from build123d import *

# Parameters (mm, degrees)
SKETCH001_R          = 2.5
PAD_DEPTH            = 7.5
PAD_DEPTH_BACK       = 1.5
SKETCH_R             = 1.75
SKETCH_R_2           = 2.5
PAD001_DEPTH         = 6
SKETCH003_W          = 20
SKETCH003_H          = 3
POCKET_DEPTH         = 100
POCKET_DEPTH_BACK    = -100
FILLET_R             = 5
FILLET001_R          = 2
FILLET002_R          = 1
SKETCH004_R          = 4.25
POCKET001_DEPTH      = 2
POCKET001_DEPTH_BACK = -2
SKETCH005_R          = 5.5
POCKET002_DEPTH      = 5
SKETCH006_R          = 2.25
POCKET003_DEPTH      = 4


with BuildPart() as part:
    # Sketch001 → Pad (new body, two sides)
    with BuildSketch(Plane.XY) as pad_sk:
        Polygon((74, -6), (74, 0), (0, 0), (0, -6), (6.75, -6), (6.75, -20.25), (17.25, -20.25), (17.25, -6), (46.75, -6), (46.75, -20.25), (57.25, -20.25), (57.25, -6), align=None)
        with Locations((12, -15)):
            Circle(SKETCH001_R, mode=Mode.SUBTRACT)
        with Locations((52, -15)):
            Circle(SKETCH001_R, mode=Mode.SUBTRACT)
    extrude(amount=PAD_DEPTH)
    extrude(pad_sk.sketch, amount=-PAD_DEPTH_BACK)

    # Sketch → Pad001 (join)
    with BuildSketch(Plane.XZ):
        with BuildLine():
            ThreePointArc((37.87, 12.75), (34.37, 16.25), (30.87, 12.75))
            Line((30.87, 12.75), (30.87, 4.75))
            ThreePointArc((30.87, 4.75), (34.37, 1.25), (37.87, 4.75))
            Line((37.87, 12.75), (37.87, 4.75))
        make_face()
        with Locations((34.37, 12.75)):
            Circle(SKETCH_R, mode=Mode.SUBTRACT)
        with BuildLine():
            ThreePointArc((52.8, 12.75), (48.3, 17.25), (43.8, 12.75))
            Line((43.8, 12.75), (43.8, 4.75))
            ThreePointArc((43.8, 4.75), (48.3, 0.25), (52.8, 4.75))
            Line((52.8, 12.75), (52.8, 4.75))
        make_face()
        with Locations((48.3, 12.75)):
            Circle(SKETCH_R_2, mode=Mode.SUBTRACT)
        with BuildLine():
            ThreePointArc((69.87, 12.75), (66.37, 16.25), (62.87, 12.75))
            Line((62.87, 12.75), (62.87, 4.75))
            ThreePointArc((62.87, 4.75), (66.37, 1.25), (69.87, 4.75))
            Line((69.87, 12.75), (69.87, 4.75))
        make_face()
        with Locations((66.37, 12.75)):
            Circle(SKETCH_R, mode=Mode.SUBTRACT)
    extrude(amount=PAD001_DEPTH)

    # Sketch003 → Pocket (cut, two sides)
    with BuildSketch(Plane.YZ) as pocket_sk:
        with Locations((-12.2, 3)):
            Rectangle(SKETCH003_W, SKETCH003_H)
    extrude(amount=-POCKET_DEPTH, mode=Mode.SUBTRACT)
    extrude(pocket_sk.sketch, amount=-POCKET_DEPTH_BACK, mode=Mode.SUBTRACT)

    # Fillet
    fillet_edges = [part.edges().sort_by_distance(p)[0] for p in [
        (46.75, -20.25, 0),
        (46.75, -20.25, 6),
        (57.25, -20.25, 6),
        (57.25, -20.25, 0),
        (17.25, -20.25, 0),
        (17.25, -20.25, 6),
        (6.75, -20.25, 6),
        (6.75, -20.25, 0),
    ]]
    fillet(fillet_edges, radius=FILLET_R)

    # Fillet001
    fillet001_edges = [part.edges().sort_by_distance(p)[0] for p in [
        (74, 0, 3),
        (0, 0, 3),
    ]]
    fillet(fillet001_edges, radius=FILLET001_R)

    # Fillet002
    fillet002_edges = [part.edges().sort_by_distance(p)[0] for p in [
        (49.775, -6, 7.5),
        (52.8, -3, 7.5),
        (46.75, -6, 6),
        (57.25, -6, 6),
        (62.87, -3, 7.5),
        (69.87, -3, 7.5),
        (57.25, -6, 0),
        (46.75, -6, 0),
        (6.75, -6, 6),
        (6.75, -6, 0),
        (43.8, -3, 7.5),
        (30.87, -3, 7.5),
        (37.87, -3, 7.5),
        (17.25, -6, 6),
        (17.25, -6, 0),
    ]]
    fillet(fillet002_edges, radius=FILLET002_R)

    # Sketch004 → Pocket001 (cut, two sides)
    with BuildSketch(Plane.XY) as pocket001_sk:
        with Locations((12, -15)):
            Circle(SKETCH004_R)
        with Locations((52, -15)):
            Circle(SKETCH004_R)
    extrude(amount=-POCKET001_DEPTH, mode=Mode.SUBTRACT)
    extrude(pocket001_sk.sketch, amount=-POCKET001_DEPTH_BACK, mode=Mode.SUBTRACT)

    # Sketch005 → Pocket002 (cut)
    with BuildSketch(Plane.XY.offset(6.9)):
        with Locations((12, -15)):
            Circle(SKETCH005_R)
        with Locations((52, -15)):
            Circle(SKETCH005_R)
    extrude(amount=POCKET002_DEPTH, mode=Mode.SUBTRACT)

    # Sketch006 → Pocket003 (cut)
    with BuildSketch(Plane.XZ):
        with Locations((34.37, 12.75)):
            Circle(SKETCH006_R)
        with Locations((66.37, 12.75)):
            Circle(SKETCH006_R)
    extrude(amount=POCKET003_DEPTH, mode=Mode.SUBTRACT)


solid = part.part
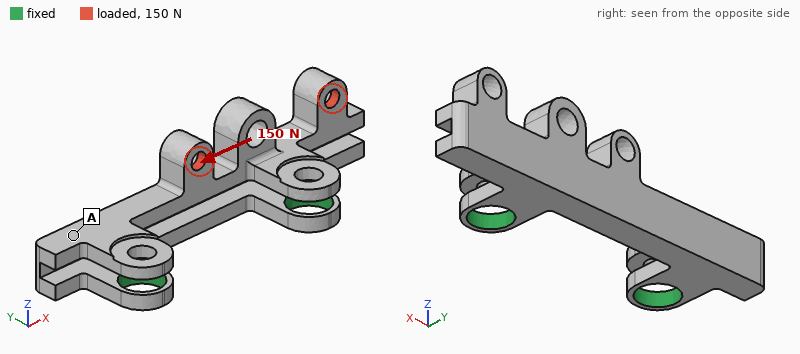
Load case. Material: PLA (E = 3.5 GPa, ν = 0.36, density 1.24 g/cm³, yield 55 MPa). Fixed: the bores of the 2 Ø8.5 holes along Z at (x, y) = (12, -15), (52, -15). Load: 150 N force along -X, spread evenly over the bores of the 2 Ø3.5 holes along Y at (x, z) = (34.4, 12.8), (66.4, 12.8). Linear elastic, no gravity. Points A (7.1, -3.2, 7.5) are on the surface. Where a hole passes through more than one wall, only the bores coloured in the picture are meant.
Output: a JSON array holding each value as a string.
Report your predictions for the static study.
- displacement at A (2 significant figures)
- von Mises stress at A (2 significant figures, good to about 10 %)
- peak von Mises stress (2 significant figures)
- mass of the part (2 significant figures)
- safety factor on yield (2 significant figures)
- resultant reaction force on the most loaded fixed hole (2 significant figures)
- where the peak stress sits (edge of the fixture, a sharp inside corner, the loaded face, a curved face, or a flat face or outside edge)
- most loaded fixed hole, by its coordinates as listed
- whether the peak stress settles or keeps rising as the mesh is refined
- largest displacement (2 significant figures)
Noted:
["0.18 mm", "3.2 MPa", "35 MPa", "6.4 g", "1.6", "93 N", "a curved face", "(12, -15)", "settles", "0.65 mm"]
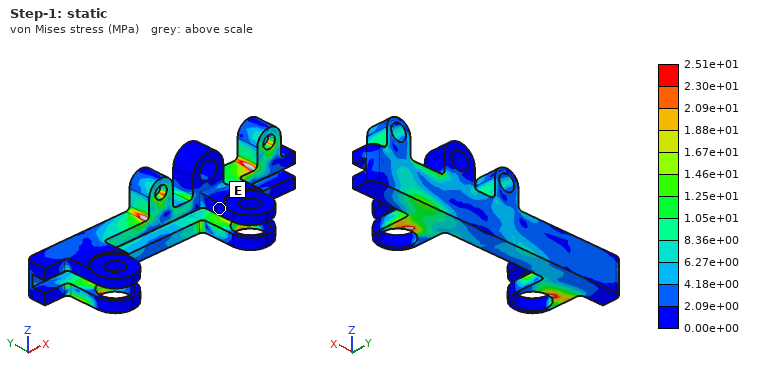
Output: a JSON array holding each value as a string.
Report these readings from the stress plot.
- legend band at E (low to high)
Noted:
["0.00e+00 to 2.09e+00 MPa"]
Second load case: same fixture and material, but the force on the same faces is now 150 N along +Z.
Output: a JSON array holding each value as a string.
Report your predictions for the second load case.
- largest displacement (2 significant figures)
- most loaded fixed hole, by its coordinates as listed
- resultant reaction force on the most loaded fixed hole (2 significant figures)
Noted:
["0.66 mm", "(52, -15)", "140 N"]
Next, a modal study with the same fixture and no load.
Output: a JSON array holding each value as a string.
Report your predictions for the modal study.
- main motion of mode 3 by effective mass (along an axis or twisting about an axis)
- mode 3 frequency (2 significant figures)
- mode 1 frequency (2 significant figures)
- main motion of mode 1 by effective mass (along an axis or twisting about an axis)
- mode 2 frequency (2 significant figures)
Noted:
["along Z", "1900 Hz", "1000 Hz", "along Y", "1600 Hz"]
